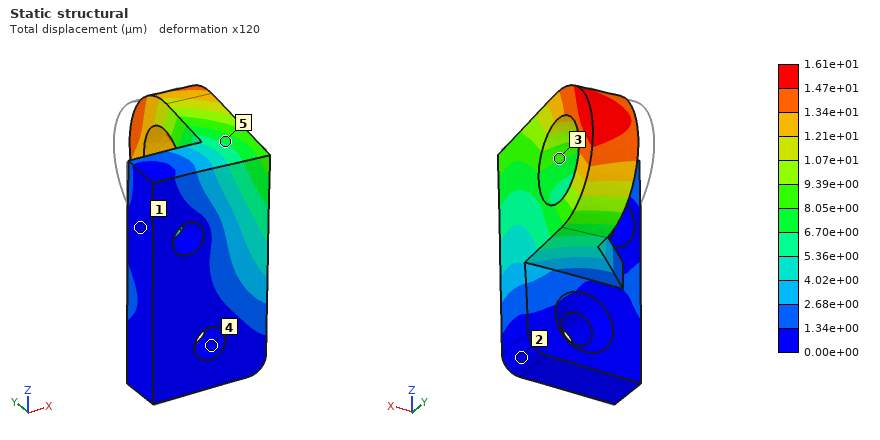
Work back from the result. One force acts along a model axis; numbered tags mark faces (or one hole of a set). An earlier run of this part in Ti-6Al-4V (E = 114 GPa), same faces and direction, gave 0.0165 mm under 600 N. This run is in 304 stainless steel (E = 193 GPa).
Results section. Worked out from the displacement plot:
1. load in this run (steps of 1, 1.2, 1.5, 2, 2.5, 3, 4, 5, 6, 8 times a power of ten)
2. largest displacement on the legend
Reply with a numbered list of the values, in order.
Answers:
1. 1 kN
2. 1.61e+01 µm
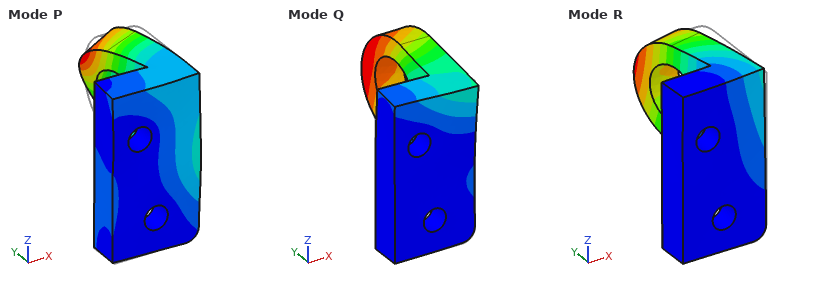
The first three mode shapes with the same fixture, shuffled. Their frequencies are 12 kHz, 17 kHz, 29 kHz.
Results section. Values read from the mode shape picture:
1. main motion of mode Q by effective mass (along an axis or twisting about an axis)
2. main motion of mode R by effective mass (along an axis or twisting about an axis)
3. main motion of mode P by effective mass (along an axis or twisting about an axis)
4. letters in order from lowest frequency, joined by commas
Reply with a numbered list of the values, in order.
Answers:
1. along Z
2. along X
3. along Y
4. R, Q, P
